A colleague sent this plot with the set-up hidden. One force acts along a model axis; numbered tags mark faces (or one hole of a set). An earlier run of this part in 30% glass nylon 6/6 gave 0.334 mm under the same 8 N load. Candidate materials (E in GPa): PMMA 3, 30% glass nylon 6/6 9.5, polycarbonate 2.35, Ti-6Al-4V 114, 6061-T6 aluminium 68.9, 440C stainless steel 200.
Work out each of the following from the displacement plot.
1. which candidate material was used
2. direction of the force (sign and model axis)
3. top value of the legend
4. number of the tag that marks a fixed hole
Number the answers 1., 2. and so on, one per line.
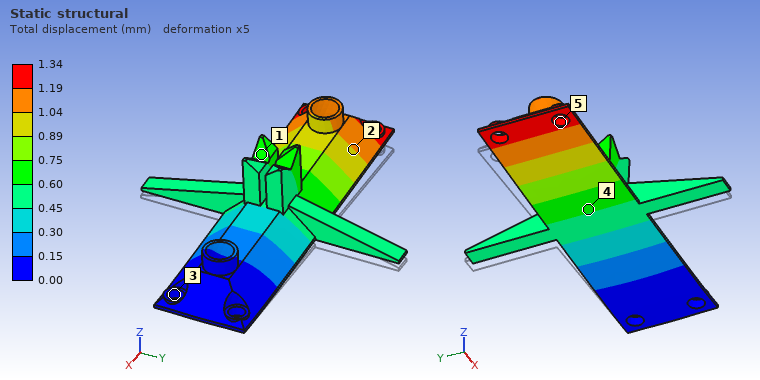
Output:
1. polycarbonate
2. +Z
3. 1.34 mm
4. 3
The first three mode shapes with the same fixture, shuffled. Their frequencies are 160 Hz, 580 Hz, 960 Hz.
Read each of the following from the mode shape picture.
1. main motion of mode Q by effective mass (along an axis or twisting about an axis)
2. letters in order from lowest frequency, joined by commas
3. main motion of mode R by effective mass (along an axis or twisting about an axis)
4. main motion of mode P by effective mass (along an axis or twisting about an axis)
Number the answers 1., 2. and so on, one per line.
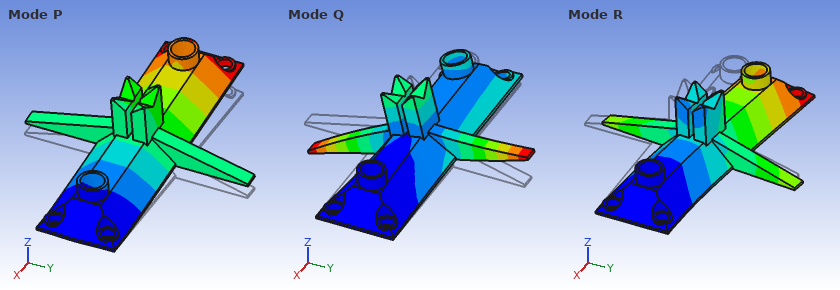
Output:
1. twisting about X
2. P, R, Q
3. along Y
4. along Z
